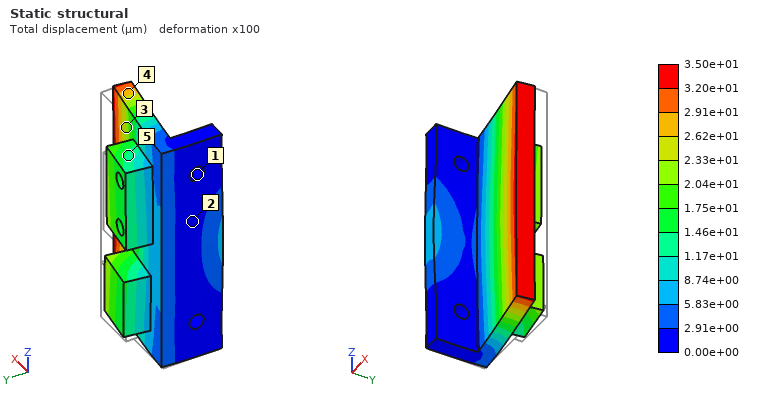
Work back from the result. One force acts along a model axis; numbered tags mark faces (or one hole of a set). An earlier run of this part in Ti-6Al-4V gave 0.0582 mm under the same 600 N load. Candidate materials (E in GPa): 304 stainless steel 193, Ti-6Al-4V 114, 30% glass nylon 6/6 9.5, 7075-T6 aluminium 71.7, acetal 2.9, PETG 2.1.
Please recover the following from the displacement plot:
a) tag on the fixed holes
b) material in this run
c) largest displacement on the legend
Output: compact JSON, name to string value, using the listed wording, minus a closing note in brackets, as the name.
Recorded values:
{"tag on the fixed holes": "1", "material in this run": "304 stainless steel", "largest displacement on the legend": "3.50e+01 µm"}
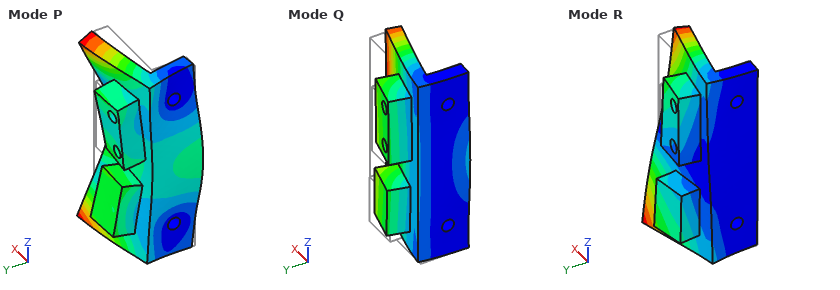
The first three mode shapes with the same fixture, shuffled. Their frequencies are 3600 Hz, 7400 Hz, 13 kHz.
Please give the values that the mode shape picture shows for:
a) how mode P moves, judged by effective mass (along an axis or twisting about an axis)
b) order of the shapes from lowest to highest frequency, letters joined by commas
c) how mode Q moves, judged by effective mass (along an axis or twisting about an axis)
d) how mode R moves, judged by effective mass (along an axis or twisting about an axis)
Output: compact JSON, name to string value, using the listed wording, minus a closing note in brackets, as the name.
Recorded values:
{"how mode P moves, judged by effective mass": "along X", "order of the shapes from lowest to highest frequency, letters joined by commas": "Q, R, P", "how mode Q moves, judged by effective mass": "along Y", "how mode R moves, judged by effective mass": "twisting about X"}
